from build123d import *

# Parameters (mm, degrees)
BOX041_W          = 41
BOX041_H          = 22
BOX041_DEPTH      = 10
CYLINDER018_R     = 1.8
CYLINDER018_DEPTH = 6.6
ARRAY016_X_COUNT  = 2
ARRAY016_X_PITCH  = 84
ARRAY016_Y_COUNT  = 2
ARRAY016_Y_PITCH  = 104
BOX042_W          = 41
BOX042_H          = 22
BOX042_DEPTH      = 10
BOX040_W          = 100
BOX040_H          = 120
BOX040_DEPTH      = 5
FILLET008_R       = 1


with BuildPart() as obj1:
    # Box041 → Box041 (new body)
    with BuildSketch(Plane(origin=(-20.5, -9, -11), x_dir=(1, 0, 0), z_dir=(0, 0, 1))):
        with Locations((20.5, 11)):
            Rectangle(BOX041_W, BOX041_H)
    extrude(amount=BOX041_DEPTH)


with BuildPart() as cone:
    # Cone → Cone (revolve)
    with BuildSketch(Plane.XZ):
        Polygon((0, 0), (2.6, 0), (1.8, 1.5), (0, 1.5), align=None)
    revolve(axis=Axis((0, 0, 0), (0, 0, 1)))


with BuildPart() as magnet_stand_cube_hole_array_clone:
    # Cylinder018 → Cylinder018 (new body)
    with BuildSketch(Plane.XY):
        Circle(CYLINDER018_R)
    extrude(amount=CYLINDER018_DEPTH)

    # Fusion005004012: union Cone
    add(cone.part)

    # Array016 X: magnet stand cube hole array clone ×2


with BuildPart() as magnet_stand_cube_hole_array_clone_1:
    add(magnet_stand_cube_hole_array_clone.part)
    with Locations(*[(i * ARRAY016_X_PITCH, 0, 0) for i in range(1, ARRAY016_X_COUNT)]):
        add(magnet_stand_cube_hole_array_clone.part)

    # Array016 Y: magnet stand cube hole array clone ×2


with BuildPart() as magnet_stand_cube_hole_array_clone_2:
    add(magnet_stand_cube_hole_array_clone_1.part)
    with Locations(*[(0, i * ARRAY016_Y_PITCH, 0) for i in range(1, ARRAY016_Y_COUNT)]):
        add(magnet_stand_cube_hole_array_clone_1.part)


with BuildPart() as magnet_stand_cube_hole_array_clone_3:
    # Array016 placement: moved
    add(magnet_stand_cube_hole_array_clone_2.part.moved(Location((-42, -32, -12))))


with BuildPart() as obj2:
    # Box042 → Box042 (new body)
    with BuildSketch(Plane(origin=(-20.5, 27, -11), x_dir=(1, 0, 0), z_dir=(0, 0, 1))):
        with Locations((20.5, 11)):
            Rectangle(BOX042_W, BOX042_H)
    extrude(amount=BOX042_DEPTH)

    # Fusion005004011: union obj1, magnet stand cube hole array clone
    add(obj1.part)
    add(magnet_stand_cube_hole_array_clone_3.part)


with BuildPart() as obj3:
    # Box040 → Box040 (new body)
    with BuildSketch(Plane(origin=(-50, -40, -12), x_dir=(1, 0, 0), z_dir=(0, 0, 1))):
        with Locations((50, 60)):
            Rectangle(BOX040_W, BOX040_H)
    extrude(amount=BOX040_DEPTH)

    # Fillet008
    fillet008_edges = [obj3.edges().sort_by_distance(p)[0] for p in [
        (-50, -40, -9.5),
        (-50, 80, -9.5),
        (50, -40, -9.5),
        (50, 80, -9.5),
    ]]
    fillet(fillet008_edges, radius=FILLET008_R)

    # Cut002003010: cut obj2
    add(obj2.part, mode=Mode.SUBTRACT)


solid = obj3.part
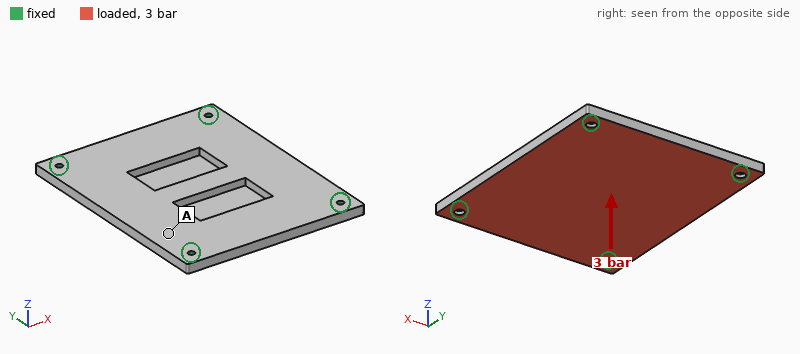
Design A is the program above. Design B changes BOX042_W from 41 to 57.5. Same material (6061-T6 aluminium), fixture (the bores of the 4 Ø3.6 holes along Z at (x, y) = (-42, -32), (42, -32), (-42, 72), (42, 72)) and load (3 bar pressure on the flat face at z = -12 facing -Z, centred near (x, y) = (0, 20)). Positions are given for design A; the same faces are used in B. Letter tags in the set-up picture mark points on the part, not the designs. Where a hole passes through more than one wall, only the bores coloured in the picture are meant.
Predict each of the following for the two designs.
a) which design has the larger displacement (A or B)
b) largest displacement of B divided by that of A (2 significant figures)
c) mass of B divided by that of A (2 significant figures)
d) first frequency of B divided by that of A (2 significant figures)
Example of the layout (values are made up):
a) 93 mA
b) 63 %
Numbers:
a) B
b) 1.1
c) 0.97
d) 1.0
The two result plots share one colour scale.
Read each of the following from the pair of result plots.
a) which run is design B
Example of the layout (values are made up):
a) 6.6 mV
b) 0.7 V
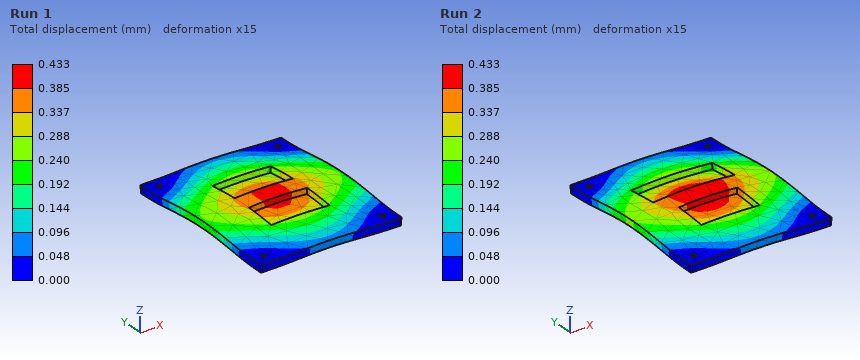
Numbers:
a) Run 2
